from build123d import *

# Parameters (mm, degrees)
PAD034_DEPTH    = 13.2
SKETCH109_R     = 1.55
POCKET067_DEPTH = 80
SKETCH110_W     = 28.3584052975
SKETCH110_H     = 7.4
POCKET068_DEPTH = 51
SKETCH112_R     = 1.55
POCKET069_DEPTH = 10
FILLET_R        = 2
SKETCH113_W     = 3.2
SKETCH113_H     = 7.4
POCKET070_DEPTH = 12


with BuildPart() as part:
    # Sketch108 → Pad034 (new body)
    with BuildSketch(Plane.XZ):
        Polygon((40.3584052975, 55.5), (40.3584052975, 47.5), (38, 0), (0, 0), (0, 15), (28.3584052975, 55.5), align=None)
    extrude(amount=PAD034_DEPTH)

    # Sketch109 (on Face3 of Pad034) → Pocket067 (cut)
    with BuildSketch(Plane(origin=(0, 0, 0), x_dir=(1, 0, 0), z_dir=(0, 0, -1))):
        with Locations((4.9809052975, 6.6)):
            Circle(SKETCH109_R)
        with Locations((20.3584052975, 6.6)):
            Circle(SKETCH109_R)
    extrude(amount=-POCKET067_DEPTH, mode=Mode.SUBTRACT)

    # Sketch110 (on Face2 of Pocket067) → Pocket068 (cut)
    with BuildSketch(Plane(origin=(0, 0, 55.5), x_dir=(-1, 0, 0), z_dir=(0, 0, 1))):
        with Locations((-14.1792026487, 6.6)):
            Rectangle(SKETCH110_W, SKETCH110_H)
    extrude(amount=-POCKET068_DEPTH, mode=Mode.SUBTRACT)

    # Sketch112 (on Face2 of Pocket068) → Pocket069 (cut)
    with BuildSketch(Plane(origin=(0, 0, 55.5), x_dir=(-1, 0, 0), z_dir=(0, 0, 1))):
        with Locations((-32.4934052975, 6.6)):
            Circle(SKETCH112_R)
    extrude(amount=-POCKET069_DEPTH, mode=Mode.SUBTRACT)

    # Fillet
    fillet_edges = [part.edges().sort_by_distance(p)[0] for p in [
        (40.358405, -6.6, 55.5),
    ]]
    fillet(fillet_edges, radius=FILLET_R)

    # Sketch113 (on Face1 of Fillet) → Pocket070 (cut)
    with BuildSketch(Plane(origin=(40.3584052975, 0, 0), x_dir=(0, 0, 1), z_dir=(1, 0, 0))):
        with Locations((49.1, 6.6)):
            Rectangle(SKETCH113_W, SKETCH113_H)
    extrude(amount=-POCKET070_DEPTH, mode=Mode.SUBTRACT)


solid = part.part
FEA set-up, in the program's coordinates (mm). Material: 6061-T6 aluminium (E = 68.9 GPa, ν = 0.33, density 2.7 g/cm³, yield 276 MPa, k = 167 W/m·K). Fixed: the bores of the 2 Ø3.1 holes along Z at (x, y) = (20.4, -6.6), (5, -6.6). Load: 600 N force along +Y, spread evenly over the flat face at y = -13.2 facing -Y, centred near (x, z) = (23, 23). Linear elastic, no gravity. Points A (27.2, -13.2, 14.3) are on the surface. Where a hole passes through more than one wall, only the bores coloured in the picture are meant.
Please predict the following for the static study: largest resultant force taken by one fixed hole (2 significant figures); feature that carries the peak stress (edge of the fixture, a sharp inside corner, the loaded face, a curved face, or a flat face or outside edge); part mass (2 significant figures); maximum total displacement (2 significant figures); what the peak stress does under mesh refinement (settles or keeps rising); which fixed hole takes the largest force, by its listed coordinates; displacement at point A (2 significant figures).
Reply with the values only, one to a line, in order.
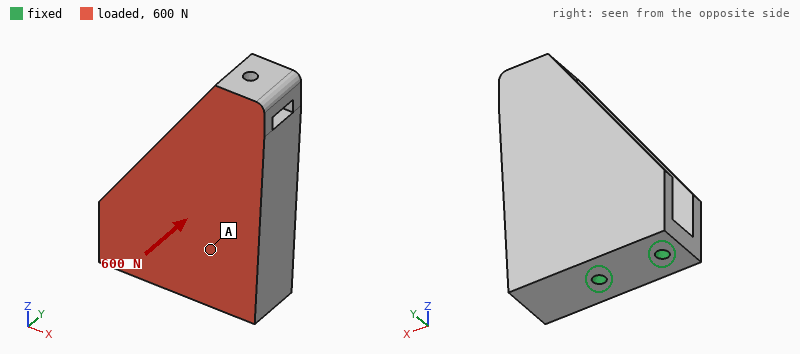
640 N
edge of the fixture
39 g
0.19 mm
keeps rising
(20.4, -6.6)
0.049 mm
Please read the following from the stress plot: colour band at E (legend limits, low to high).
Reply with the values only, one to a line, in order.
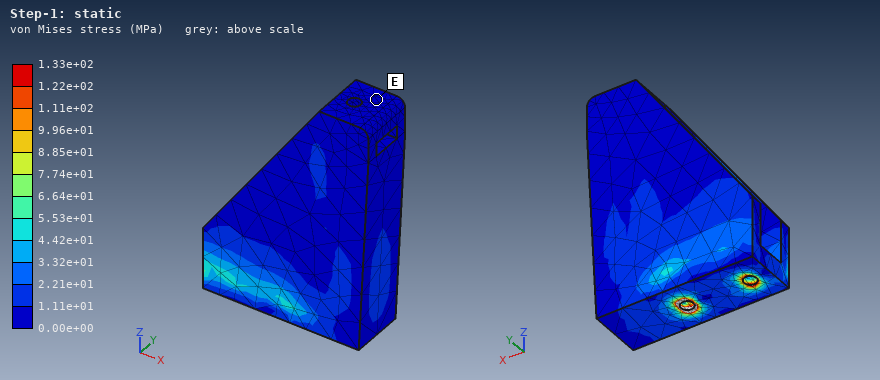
0.00e+00 to 1.11e+01 MPa
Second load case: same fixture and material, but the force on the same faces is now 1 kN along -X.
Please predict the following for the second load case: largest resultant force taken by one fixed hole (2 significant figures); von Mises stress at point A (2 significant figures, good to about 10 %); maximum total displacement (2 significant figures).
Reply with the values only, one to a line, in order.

1.3 kN
14 MPa
66 µm
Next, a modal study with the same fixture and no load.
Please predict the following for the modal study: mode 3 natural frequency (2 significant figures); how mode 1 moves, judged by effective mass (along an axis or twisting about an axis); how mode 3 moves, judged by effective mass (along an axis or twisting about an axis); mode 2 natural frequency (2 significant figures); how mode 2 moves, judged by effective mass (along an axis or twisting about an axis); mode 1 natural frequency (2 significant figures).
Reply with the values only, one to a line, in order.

7300 Hz
along Y
twisting about Z
4000 Hz
along X
1900 Hz
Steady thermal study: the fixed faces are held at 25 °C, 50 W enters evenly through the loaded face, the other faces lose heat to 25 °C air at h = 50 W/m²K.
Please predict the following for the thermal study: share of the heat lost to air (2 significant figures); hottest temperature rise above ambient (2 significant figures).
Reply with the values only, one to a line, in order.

12 %
33 K
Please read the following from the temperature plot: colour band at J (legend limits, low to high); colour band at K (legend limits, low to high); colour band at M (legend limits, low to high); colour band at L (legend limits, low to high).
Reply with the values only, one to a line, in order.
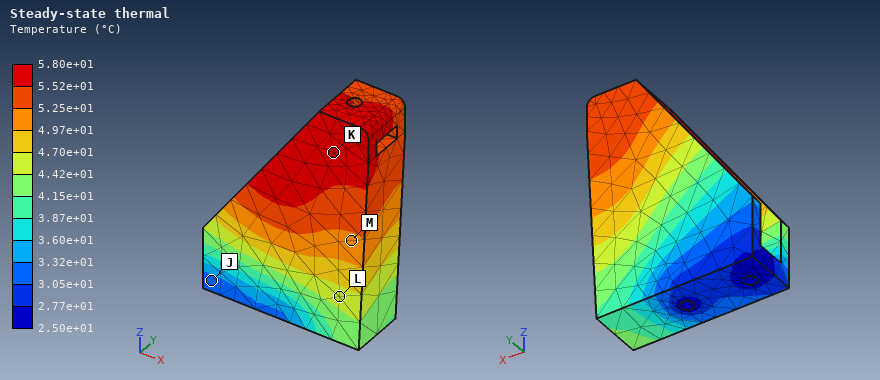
3.05e+01 to 3.32e+01 °C
5.52e+01 to 5.80e+01 °C
4.97e+01 to 5.25e+01 °C
4.42e+01 to 4.70e+01 °C
